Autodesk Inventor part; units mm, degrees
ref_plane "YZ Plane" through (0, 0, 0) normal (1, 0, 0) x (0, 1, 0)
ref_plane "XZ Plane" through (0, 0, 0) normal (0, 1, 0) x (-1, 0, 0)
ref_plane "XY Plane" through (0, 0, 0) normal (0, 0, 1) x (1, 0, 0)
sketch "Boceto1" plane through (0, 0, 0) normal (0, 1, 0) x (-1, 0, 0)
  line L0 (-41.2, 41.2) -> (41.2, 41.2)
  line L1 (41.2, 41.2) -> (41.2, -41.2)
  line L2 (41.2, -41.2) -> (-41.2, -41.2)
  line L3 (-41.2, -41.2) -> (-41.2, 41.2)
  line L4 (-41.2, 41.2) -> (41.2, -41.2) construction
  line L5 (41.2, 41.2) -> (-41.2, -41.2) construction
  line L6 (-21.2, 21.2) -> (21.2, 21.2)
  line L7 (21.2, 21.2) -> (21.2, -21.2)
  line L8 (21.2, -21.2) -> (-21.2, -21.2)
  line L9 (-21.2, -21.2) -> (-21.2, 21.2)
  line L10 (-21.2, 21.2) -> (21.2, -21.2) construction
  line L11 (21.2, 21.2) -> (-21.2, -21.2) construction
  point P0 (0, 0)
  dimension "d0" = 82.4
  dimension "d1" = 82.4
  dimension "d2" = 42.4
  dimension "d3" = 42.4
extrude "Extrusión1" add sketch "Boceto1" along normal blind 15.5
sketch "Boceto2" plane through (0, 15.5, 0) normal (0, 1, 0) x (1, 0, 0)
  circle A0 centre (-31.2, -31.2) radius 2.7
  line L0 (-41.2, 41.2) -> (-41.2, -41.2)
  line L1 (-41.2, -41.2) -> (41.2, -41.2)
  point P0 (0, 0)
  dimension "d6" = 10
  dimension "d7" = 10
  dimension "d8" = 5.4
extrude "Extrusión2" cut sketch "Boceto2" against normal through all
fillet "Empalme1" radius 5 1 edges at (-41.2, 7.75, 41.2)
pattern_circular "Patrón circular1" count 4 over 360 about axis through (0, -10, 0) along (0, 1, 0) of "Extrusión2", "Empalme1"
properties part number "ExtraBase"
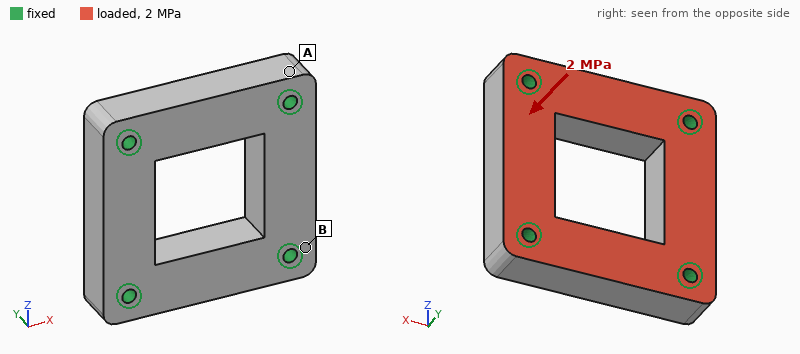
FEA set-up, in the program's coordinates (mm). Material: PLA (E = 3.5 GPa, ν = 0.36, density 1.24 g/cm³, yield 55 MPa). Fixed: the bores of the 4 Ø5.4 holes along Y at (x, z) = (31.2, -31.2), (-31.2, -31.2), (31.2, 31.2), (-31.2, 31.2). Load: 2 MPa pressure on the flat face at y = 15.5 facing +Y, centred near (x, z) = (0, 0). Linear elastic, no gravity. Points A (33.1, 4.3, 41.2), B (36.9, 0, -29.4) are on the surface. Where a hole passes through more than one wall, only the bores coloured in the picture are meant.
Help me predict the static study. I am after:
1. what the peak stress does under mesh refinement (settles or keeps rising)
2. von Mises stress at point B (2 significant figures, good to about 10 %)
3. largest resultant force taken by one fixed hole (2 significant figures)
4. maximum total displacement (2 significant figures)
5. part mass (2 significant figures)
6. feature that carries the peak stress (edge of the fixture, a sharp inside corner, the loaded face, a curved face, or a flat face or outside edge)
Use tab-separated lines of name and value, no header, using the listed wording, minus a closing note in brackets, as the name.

what the peak stress does under mesh refinement	keeps rising
von Mises stress at point B	8.7 MPa
largest resultant force taken by one fixed hole	2.4 kN
maximum total displacement	0.17 mm
part mass	94 g
feature that carries the peak stress	edge of the fixture
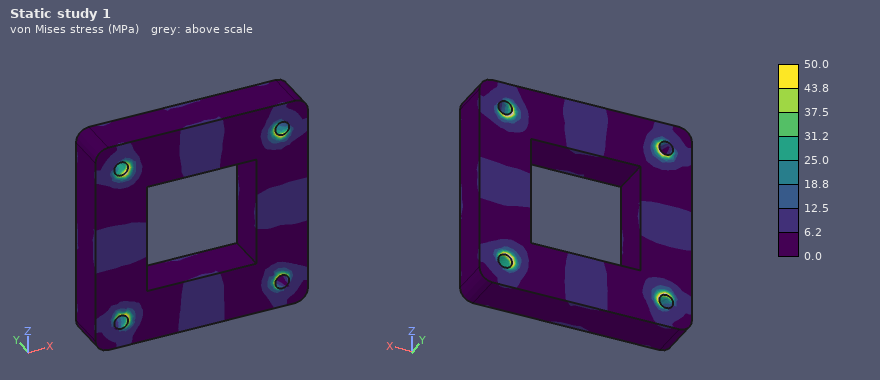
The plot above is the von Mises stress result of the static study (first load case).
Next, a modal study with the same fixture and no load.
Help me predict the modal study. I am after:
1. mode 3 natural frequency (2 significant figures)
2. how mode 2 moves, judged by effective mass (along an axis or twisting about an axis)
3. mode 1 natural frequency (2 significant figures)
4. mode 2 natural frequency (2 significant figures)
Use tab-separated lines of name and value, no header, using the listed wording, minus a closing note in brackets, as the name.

mode 3 natural frequency	5100 Hz
how mode 2 moves, judged by effective mass	along Y
mode 1 natural frequency	4300 Hz
mode 2 natural frequency	4700 Hz
